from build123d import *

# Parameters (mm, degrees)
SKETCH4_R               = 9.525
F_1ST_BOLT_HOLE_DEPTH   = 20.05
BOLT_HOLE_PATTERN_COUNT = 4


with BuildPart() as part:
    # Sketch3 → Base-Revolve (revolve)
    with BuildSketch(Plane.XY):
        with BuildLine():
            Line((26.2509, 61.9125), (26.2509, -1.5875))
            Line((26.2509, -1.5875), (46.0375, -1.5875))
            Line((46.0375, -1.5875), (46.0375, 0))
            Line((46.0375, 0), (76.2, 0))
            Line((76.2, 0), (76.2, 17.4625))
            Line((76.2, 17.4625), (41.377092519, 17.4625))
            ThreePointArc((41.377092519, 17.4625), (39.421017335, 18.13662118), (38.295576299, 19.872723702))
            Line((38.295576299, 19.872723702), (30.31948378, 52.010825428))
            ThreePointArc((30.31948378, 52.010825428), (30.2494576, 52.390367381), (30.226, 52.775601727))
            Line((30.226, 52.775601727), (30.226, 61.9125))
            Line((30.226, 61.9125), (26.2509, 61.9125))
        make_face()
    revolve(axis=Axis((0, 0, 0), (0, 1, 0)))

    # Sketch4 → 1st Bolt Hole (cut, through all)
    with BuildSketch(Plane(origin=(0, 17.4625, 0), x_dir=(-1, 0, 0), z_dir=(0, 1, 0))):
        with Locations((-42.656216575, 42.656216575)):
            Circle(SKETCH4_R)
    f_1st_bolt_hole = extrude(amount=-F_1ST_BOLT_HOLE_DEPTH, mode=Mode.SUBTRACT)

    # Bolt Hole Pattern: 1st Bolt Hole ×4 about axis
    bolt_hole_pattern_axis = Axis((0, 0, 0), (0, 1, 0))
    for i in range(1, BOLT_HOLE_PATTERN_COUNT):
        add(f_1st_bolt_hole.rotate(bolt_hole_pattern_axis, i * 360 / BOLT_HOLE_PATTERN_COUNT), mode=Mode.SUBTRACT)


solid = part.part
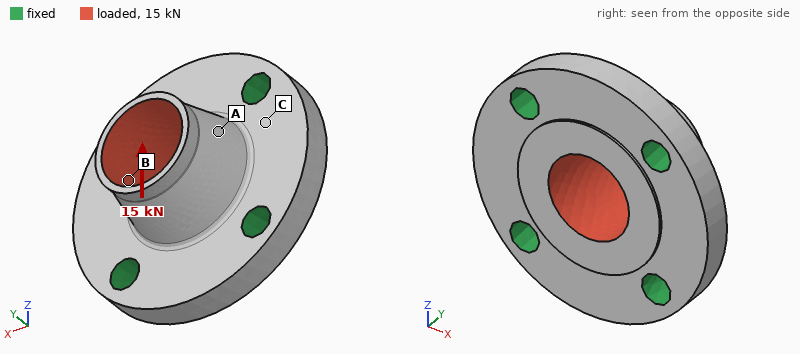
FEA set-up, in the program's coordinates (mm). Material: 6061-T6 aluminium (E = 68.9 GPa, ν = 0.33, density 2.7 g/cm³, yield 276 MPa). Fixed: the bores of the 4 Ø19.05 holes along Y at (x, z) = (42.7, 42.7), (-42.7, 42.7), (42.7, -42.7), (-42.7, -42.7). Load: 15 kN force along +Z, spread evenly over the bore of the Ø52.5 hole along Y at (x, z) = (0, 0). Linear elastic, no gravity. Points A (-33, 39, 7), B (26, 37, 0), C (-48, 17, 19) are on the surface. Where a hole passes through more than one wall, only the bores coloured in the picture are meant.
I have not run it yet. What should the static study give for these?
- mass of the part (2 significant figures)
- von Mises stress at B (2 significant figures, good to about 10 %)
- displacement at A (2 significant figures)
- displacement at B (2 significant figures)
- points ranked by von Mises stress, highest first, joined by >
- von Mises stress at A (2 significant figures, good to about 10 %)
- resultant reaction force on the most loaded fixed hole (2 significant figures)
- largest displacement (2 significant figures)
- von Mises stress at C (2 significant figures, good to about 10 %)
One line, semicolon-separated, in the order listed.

890 g; 16 MPa; 10 µm; 10 µm; B > A > C; 9.8 MPa; 4.4 kN; 25 µm; 4.2 MPa
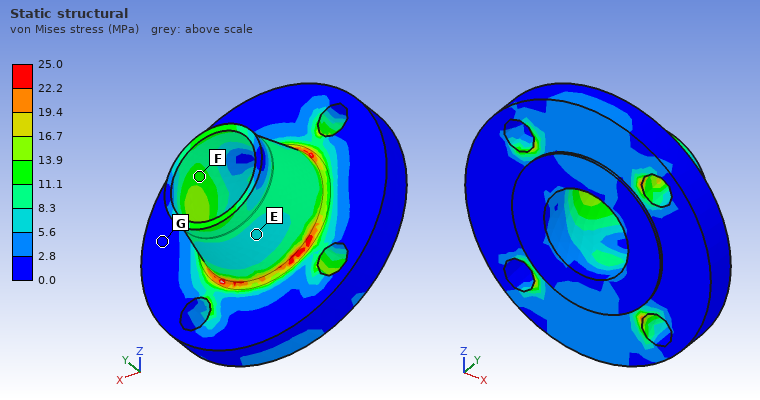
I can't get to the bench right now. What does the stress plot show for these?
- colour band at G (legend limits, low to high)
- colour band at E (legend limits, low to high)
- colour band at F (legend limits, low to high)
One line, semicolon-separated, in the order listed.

0.0 to 2.8 MPa; 5.6 to 8.3 MPa; 11.1 to 13.9 MPa
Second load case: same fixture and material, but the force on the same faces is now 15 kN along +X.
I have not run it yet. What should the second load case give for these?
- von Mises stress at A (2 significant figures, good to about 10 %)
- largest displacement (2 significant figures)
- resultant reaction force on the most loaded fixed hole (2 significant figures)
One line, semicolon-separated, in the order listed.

6.7 MPa; 25 µm; 4.4 kN
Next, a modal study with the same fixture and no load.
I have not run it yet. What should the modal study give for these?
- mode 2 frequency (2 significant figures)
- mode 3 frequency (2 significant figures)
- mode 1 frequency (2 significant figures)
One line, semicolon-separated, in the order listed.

9700 Hz; 9700 Hz; 8800 Hz
